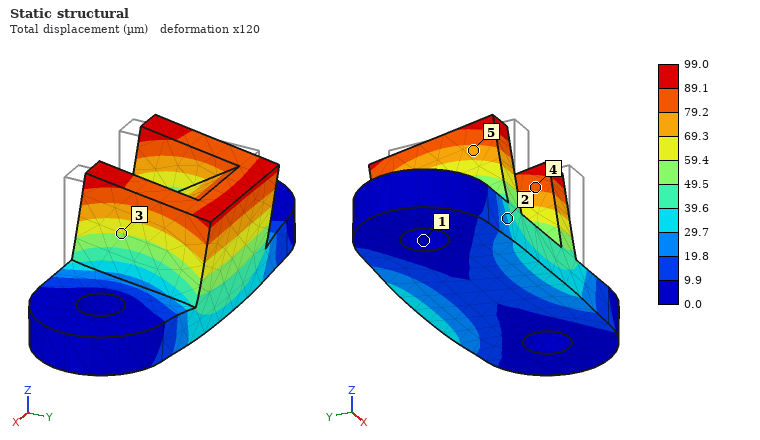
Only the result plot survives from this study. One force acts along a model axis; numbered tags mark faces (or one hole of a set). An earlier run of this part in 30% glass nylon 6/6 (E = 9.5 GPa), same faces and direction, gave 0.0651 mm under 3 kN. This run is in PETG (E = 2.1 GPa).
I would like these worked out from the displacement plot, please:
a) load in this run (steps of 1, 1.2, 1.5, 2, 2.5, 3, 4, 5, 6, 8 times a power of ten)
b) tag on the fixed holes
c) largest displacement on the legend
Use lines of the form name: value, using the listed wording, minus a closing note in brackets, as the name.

load in this run: 1 kN
tag on the fixed holes: 1
largest displacement on the legend: 99.0 µm
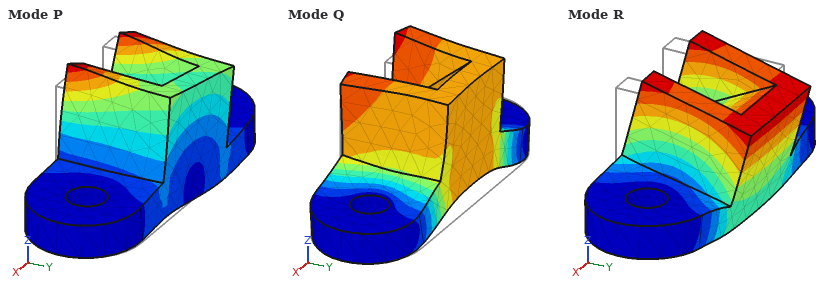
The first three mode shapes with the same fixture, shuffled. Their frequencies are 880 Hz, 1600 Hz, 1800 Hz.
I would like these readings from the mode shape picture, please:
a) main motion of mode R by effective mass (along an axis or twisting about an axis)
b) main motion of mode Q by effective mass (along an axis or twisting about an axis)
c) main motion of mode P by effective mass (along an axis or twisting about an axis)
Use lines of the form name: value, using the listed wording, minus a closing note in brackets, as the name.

main motion of mode R by effective mass: along Y
main motion of mode Q by effective mass: along Z
main motion of mode P by effective mass: along X
